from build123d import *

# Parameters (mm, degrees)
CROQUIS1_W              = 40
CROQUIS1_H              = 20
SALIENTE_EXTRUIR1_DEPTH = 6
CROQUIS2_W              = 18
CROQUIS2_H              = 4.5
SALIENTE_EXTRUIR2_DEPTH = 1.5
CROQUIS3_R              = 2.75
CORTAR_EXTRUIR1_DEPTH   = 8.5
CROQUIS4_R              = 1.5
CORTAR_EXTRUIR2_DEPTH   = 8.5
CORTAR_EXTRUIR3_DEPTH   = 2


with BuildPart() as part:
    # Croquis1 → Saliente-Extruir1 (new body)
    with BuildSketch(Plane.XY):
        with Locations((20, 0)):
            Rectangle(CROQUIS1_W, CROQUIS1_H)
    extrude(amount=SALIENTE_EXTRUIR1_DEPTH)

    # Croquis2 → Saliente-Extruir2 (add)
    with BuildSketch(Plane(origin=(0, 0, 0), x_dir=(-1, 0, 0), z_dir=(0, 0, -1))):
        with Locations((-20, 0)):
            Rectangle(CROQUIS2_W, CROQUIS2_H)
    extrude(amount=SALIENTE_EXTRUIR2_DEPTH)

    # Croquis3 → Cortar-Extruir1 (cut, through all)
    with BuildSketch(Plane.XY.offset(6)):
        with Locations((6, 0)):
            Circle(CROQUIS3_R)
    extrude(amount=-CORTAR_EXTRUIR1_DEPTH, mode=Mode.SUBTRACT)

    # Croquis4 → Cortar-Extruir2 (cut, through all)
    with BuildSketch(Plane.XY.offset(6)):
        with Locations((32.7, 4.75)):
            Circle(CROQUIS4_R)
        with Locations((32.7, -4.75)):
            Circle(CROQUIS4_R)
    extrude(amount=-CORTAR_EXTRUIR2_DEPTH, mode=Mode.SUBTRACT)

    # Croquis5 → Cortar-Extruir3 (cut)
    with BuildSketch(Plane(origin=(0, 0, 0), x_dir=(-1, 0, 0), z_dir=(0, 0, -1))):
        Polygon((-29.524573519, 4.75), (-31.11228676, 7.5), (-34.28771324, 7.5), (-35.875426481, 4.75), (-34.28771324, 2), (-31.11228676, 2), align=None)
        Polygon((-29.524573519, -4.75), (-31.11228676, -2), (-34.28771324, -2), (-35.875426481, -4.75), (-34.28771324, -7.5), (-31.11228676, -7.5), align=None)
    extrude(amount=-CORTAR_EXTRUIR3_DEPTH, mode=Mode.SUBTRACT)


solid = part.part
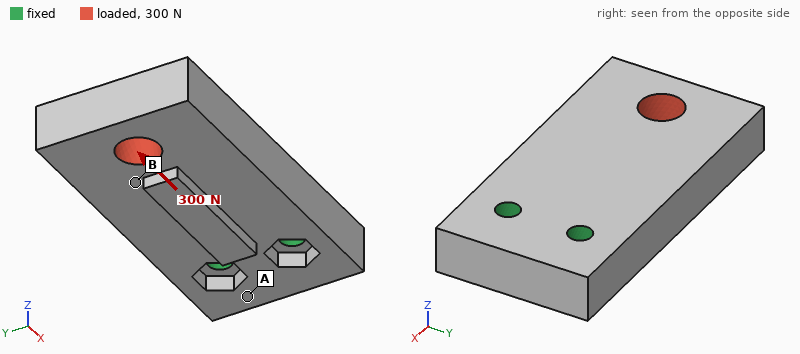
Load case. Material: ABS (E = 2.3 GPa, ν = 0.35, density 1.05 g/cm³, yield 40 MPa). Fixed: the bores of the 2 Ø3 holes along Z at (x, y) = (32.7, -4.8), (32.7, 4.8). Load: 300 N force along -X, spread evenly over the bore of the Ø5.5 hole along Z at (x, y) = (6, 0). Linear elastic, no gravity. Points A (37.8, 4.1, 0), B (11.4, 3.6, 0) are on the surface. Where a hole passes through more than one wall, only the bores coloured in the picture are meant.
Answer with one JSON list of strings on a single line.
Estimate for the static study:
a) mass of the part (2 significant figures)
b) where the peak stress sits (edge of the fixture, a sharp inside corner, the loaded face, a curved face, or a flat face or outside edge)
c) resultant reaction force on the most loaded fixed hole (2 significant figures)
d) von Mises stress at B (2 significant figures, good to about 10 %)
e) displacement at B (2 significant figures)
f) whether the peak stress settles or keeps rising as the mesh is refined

["4.8 g", "edge of the fixture", "150 N", "3.4 MPa", "52 µm", "keeps rising"]
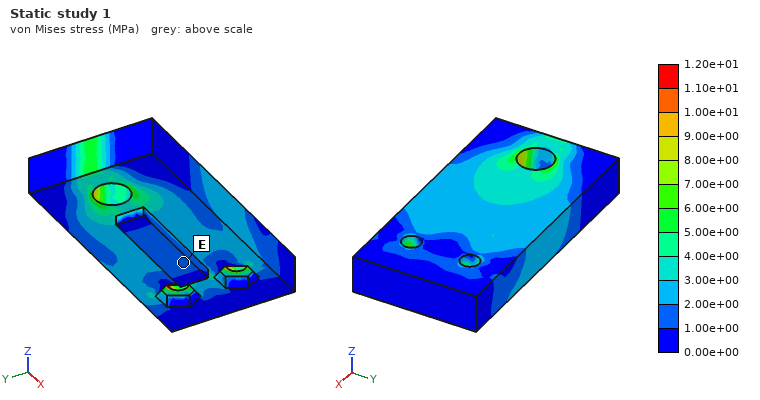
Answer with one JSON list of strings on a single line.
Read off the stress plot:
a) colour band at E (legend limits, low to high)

["1.00e+00 to 2.00e+00 MPa"]
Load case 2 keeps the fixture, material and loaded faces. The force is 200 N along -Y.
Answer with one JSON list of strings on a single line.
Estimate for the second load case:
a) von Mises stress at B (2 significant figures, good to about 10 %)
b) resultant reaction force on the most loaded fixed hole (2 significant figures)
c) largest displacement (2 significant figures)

["3.3 MPa", "480 N", "0.37 mm"]
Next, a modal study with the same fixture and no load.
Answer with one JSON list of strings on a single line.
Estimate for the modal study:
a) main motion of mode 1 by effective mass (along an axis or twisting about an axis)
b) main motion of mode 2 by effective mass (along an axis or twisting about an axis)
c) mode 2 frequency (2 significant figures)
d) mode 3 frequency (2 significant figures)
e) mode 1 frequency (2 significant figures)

["along Z", "along Y", "3100 Hz", "3800 Hz", "1200 Hz"]
